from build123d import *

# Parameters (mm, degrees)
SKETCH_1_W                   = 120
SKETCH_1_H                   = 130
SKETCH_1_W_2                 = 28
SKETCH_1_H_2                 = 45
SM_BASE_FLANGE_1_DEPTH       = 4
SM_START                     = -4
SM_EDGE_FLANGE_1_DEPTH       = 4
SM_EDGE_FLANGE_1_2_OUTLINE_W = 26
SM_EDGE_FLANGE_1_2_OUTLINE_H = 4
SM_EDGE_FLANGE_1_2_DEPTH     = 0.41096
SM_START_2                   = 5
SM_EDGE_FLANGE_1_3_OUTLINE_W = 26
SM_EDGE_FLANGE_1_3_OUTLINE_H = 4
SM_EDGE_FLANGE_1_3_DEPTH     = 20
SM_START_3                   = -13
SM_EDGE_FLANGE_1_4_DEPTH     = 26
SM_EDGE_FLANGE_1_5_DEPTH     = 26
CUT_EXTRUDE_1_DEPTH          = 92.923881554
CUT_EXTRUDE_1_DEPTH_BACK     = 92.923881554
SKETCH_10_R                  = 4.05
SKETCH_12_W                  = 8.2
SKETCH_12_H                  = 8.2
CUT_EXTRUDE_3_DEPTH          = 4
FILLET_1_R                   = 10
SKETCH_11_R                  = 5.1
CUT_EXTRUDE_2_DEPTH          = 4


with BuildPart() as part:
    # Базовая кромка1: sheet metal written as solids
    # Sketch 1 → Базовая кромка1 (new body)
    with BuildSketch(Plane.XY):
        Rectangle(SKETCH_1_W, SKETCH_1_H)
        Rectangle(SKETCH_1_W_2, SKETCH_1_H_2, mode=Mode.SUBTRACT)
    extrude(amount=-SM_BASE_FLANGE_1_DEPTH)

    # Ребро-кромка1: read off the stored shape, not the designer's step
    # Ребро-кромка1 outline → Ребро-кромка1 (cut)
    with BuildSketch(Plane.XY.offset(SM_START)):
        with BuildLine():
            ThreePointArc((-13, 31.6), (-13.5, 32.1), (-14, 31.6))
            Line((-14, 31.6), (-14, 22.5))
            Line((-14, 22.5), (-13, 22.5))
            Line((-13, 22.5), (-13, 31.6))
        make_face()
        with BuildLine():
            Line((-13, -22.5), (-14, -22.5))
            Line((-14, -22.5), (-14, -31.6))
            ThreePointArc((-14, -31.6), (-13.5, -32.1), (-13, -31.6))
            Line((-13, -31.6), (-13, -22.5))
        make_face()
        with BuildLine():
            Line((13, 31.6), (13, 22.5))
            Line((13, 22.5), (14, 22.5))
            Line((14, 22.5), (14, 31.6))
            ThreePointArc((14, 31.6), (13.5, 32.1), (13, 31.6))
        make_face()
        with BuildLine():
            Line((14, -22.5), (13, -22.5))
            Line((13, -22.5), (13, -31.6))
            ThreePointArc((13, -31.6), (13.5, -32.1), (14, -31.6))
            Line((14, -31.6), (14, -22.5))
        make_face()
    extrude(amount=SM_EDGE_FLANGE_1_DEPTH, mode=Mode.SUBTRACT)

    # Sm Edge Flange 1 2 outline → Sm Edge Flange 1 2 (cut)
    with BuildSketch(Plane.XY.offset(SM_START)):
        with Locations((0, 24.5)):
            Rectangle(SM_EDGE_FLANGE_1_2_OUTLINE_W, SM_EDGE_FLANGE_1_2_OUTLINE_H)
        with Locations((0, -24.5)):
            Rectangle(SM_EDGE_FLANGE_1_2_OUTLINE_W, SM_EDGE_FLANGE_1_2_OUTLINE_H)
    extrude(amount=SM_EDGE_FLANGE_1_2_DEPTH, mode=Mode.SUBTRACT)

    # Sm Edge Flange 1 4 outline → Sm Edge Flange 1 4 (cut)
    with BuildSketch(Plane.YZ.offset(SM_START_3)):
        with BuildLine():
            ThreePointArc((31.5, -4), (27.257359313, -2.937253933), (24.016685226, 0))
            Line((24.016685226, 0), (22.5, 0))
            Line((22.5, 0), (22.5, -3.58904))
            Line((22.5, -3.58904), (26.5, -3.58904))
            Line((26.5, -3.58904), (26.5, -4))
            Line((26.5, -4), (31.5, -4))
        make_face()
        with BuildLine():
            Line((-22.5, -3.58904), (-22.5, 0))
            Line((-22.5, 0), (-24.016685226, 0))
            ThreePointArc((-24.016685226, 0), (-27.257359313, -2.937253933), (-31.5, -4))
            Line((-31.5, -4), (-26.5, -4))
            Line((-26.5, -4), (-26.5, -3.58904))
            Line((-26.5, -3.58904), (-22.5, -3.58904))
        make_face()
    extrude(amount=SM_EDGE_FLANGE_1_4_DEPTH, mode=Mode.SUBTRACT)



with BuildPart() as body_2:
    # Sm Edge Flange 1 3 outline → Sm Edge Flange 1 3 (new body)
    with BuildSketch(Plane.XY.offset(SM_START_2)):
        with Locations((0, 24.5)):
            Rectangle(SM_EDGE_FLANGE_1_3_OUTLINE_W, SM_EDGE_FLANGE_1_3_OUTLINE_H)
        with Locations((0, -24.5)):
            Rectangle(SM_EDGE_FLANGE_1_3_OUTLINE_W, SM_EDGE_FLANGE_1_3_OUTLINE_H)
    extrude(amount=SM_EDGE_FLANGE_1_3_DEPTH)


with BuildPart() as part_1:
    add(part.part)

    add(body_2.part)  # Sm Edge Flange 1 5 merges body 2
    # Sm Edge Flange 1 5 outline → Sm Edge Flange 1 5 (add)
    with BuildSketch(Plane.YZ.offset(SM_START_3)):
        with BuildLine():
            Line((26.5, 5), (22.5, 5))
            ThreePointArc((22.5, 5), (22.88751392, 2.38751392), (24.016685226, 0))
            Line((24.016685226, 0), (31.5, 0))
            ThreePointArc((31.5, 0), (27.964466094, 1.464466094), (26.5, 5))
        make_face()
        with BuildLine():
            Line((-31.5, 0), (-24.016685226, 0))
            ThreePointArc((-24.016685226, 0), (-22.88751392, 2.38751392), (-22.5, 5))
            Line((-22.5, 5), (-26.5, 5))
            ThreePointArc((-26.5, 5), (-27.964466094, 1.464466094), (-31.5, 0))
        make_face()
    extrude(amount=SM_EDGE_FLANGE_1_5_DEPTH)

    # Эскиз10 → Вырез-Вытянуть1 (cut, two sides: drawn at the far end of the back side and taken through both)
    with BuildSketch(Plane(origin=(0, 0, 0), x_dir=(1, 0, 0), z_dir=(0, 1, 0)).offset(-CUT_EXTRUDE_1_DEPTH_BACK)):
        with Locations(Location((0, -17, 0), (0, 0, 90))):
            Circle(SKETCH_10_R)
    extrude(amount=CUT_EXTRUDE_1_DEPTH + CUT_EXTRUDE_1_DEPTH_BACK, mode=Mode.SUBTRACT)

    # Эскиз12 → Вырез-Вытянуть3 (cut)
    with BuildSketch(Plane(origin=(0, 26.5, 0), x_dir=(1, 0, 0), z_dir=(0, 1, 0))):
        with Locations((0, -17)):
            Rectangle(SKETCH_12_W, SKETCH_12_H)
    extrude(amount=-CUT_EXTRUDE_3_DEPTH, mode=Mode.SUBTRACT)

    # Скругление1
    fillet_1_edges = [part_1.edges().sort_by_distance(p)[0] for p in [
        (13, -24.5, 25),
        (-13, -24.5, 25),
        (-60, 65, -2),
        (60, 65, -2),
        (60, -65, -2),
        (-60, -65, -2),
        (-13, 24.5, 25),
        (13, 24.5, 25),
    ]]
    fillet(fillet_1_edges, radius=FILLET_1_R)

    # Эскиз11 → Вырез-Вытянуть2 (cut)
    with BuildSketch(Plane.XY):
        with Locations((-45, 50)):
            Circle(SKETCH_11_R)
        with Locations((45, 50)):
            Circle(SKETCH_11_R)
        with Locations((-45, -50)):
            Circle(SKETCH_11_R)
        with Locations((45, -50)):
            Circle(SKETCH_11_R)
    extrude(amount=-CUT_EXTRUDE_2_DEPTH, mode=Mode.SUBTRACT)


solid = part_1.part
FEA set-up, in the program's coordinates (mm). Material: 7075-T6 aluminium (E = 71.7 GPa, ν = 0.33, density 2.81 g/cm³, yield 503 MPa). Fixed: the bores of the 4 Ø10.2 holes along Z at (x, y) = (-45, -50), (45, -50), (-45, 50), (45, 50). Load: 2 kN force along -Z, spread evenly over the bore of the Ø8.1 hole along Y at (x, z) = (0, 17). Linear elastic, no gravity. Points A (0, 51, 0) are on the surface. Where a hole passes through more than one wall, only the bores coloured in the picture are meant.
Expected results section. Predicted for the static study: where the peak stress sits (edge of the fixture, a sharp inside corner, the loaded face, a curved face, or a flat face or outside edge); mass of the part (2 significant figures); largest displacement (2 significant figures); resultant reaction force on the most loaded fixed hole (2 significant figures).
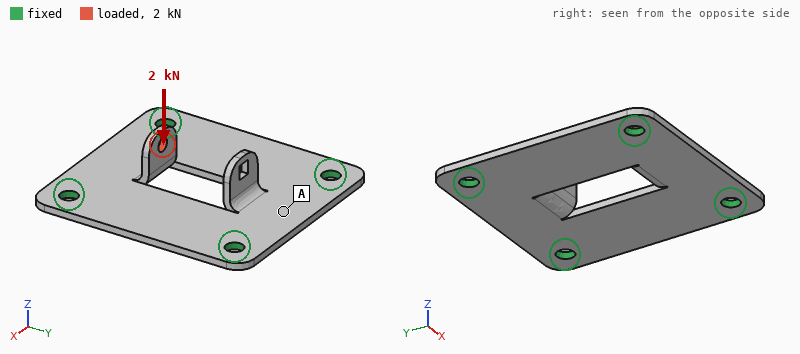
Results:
a curved face
170 g
1.5 mm
860 N
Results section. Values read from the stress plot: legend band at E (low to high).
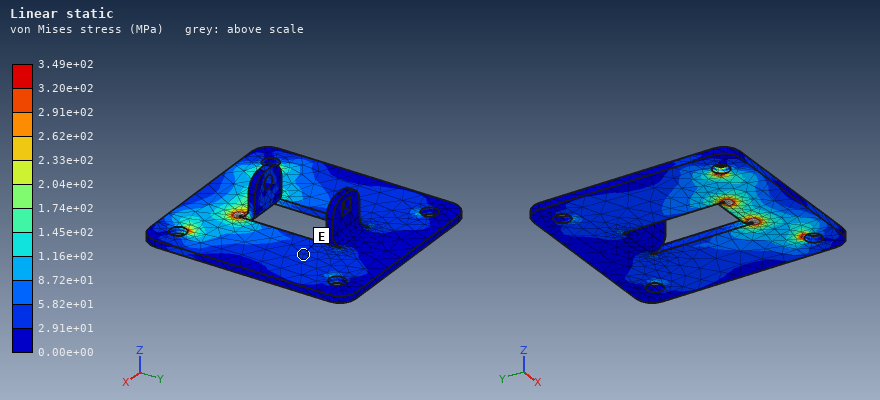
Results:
2.91e+01 to 5.82e+01 MPa
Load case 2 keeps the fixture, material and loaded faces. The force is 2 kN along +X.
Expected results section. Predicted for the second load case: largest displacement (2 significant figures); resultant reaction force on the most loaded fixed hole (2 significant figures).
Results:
0.75 mm
1.3 kN
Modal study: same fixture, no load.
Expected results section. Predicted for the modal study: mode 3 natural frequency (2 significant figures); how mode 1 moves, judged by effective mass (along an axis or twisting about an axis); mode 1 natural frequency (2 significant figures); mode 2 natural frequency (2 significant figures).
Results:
2300 Hz
along Z
1600 Hz
2300 Hz
